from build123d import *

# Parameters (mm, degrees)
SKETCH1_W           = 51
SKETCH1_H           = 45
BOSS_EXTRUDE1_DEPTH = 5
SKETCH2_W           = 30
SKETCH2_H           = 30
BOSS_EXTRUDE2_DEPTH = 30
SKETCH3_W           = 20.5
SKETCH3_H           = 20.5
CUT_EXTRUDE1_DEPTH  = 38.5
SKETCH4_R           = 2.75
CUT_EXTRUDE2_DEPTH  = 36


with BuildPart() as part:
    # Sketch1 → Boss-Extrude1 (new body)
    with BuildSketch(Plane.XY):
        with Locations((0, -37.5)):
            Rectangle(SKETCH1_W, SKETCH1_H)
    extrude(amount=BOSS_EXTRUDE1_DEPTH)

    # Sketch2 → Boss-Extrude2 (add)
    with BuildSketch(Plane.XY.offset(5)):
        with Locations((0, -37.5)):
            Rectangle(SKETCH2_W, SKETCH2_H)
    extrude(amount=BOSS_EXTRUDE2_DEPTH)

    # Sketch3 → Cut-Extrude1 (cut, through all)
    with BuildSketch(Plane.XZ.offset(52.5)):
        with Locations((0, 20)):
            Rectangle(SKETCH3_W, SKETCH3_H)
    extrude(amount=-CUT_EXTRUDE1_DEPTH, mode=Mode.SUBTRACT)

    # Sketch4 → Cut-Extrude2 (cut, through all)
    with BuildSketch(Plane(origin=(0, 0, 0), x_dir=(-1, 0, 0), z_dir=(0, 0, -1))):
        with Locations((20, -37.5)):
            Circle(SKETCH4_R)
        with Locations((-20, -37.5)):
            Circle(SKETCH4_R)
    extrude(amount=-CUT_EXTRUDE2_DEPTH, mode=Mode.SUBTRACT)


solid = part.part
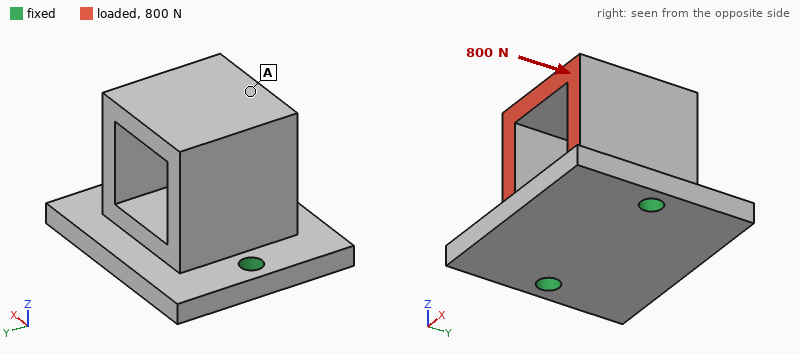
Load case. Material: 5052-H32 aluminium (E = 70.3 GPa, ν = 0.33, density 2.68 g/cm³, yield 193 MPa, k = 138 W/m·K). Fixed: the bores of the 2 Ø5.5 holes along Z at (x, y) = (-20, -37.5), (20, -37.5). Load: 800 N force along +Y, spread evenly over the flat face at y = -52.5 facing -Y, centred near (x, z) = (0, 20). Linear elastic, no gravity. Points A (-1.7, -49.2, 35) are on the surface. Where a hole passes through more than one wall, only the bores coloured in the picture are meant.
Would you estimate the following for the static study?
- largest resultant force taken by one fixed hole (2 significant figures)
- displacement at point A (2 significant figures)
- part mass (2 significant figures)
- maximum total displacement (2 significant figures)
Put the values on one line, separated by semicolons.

400 N; 49 µm; 69 g; 51 µm
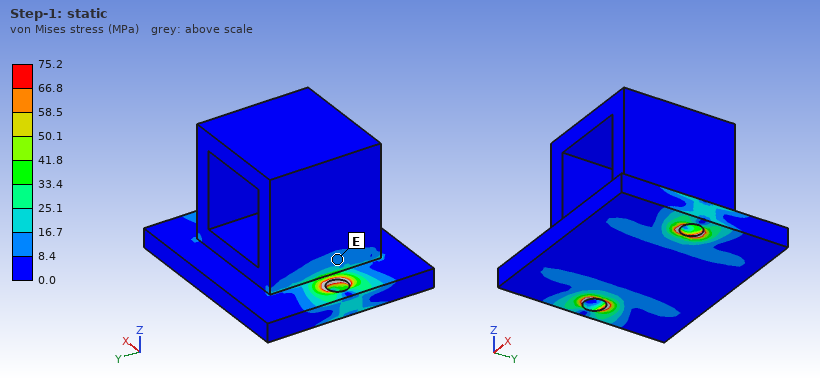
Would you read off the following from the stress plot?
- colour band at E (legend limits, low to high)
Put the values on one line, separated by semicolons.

8.4 to 16.7 MPa
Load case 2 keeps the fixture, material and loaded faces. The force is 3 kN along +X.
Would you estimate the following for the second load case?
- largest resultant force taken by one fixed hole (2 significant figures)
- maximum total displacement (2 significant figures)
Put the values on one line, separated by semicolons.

2.4 kN; 0.12 mm
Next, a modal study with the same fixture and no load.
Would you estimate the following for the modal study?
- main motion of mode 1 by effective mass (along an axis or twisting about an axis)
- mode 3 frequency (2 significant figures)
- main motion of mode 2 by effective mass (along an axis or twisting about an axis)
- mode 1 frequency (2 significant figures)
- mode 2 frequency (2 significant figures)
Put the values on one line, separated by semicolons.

along Y; 10 kHz; along X; 3300 Hz; 5300 Hz
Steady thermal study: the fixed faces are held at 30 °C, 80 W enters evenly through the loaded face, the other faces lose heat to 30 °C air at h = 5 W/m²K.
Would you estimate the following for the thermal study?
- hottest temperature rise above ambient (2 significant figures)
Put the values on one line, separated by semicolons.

60 K
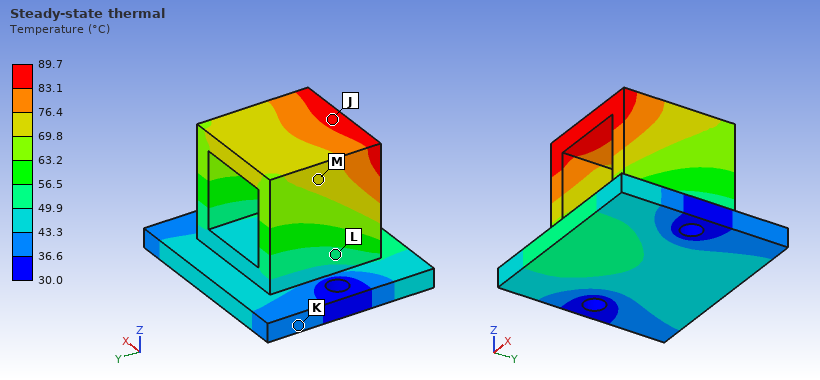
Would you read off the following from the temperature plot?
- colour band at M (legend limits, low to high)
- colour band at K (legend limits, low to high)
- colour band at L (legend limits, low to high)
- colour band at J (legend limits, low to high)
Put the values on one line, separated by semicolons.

69.8 to 76.4 °C; 36.6 to 43.3 °C; 49.9 to 56.5 °C; 83.1 to 89.7 °C
